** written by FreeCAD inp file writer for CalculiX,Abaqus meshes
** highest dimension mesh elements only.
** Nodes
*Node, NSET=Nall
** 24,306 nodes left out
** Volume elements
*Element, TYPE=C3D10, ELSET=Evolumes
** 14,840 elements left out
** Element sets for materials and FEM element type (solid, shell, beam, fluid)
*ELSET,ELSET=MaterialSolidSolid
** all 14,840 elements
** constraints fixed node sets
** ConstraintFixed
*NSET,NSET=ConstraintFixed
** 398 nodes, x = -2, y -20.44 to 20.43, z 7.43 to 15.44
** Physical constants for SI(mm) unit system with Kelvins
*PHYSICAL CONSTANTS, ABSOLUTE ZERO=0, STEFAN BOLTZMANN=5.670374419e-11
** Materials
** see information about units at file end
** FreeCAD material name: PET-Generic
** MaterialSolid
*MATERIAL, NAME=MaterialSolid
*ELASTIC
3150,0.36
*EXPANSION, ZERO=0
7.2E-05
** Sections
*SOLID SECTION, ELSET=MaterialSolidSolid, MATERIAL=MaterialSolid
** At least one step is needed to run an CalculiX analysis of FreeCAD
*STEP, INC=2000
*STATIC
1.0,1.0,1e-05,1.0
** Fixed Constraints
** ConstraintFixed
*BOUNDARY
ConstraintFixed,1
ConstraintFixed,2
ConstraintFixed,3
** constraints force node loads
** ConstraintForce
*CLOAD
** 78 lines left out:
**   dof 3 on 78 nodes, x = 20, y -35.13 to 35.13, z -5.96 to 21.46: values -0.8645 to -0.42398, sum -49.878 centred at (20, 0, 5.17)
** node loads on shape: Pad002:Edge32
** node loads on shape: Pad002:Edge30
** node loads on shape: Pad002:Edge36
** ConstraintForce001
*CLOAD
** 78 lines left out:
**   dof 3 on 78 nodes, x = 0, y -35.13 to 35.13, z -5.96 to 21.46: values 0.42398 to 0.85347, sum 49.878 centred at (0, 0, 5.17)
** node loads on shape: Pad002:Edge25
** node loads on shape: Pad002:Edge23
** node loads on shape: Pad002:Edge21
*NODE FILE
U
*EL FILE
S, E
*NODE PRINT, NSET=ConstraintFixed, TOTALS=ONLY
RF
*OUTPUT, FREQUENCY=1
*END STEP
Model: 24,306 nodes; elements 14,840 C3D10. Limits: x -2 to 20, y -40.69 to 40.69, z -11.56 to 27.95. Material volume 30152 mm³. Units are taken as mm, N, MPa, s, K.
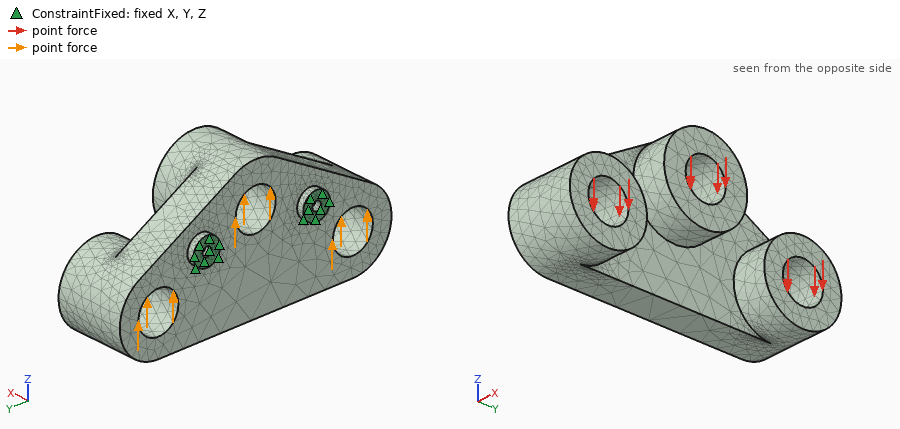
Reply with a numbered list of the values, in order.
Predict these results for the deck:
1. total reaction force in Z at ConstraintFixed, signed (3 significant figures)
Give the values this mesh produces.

1. -3.16e-06 N
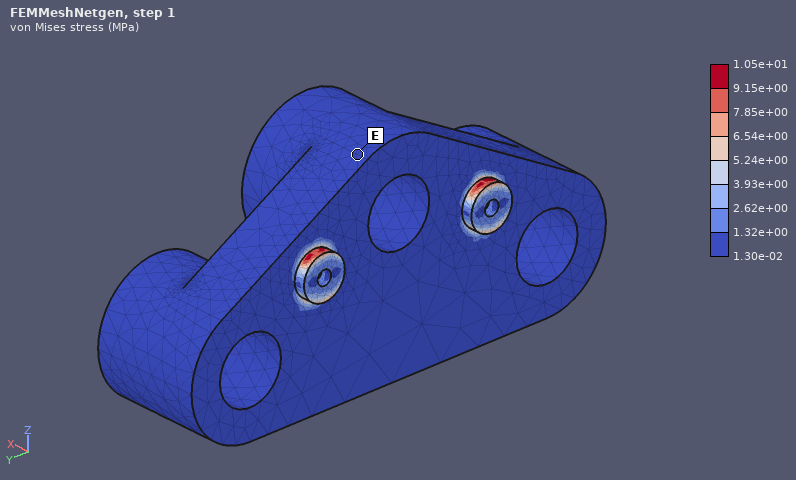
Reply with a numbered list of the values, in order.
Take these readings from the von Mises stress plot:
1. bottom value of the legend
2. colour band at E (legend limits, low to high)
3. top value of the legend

1. 1.30e-02 MPa
2. 1.30e-02 to 1.32e+00 MPa
3. 1.05e+01 MPa
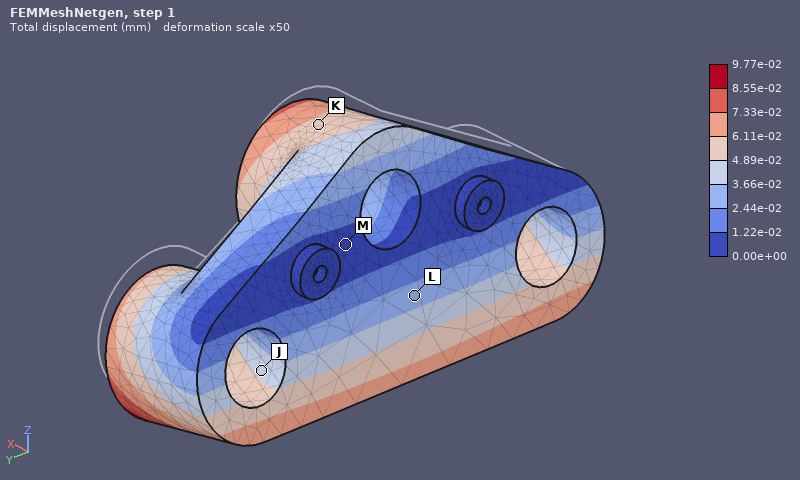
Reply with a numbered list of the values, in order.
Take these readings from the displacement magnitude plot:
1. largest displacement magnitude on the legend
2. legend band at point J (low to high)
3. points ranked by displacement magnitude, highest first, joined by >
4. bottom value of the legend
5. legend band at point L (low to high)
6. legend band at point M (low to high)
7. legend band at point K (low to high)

1. 9.77e-02 mm
2. 3.66e-02 to 4.89e-02 mm
3. K > J > L > M
4. 0.00e+00 mm
5. 2.44e-02 to 3.66e-02 mm
6. 0.00e+00 to 1.22e-02 mm
7. 4.89e-02 to 6.11e-02 mm
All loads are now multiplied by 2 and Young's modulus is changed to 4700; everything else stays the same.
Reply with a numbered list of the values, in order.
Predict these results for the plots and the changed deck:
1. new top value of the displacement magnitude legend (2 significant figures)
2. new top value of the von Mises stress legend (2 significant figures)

1. 0.13 mm
2. 21 MPa
